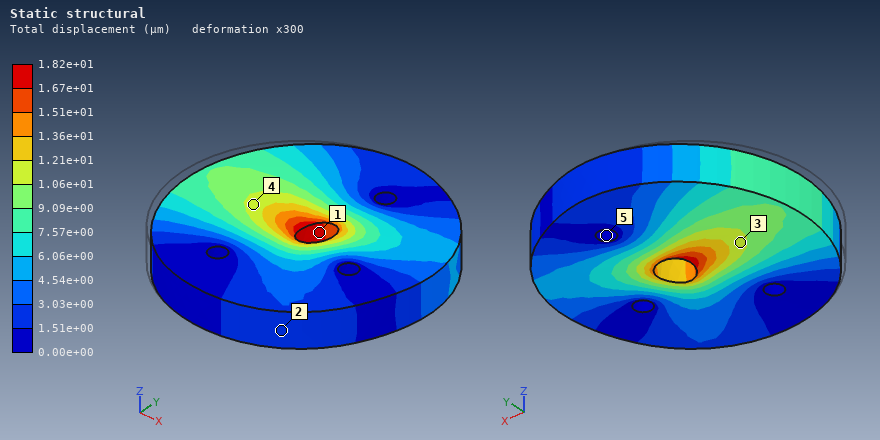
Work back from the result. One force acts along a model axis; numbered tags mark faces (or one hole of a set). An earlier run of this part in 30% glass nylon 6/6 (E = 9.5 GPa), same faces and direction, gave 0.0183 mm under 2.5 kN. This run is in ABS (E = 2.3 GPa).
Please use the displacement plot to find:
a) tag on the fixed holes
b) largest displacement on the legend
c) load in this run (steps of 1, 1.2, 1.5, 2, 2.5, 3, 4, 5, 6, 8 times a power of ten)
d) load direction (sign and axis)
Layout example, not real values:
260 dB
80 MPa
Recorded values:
5
1.82e+01 µm
600 N
+X
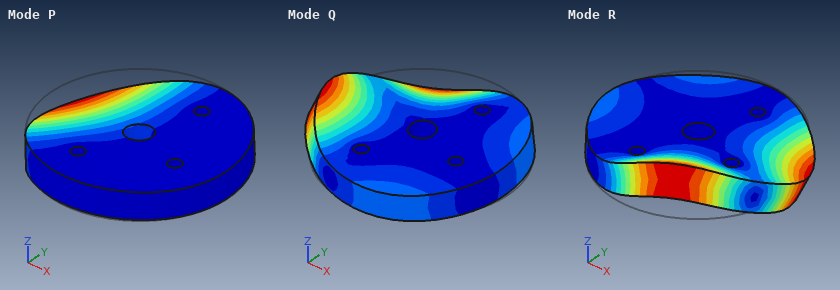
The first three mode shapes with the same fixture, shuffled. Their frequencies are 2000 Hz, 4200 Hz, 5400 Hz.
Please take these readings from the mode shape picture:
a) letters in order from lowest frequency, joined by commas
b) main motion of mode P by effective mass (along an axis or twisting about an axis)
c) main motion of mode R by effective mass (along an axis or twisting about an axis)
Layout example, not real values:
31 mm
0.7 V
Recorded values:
P, Q, R
along Z
twisting about X
